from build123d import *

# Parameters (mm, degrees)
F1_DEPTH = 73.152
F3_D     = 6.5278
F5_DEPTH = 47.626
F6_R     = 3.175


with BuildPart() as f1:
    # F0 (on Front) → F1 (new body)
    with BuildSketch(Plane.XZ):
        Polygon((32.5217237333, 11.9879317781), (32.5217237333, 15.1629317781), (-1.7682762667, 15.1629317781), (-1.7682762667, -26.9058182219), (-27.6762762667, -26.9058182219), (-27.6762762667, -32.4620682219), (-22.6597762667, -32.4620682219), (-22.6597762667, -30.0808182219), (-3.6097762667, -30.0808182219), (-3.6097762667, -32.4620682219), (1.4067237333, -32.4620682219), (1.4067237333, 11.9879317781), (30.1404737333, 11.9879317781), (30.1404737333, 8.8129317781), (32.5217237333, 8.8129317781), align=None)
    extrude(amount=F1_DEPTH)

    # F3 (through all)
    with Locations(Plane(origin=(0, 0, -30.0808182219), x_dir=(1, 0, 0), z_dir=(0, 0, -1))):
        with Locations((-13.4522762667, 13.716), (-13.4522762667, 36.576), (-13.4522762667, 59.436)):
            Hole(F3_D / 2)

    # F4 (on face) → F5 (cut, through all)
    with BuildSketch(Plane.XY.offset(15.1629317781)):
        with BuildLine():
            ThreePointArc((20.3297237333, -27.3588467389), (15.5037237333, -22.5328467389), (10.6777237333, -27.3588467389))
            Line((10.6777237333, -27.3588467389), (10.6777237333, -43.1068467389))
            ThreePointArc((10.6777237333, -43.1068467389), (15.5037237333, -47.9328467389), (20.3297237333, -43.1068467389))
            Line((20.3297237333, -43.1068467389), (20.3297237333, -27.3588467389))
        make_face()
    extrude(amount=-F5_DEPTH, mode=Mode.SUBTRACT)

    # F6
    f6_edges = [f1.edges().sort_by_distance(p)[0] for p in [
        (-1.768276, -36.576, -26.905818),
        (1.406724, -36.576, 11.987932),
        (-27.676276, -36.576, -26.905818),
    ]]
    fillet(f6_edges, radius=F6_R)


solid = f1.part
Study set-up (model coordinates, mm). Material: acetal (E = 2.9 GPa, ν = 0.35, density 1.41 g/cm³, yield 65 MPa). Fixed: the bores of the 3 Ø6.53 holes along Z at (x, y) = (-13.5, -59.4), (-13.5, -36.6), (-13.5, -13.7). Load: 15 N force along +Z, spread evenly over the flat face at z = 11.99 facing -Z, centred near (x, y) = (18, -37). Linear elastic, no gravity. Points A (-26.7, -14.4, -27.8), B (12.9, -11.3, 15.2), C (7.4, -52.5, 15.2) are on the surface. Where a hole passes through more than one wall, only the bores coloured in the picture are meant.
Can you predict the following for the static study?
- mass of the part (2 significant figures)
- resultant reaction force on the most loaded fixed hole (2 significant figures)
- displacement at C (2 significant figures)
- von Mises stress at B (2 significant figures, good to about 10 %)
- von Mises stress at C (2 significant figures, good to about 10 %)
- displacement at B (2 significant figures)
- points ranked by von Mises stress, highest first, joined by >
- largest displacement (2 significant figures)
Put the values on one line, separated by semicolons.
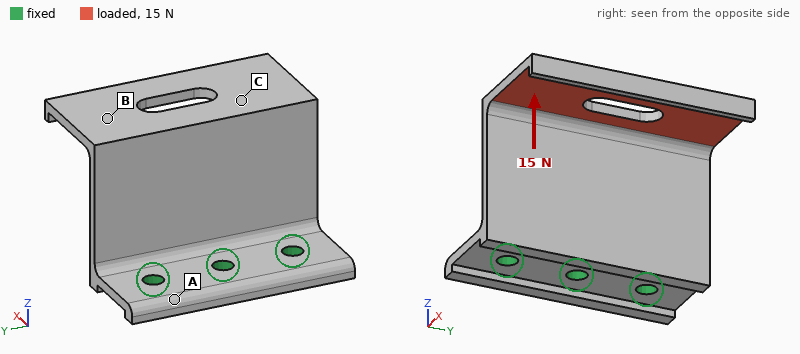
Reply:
36 g; 5.3 N; 0.66 mm; 0.91 MPa; 1.5 MPa; 0.72 mm; C > B > A; 1.1 mm
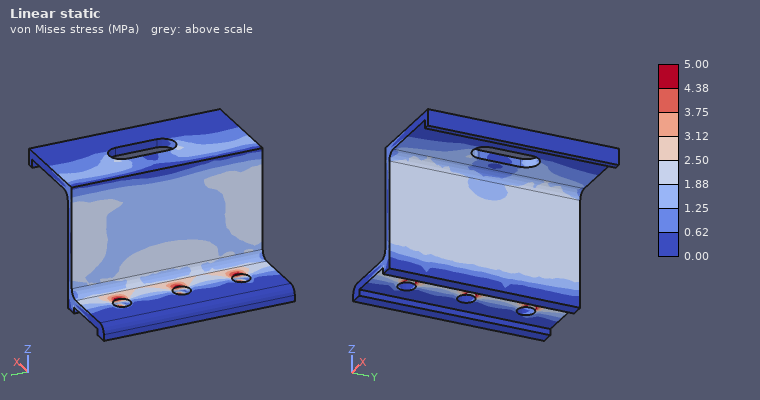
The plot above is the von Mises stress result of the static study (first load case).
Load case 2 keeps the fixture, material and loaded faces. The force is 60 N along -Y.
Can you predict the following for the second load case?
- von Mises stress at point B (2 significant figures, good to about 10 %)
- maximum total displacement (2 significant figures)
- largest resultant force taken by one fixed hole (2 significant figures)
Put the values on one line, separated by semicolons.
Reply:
1.9 MPa; 1.2 mm; 64 N
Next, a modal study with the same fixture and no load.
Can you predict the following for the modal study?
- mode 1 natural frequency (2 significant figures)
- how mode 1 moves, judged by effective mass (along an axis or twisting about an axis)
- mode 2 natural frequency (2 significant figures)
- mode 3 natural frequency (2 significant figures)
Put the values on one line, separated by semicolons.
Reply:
140 Hz; along X; 300 Hz; 500 Hz
